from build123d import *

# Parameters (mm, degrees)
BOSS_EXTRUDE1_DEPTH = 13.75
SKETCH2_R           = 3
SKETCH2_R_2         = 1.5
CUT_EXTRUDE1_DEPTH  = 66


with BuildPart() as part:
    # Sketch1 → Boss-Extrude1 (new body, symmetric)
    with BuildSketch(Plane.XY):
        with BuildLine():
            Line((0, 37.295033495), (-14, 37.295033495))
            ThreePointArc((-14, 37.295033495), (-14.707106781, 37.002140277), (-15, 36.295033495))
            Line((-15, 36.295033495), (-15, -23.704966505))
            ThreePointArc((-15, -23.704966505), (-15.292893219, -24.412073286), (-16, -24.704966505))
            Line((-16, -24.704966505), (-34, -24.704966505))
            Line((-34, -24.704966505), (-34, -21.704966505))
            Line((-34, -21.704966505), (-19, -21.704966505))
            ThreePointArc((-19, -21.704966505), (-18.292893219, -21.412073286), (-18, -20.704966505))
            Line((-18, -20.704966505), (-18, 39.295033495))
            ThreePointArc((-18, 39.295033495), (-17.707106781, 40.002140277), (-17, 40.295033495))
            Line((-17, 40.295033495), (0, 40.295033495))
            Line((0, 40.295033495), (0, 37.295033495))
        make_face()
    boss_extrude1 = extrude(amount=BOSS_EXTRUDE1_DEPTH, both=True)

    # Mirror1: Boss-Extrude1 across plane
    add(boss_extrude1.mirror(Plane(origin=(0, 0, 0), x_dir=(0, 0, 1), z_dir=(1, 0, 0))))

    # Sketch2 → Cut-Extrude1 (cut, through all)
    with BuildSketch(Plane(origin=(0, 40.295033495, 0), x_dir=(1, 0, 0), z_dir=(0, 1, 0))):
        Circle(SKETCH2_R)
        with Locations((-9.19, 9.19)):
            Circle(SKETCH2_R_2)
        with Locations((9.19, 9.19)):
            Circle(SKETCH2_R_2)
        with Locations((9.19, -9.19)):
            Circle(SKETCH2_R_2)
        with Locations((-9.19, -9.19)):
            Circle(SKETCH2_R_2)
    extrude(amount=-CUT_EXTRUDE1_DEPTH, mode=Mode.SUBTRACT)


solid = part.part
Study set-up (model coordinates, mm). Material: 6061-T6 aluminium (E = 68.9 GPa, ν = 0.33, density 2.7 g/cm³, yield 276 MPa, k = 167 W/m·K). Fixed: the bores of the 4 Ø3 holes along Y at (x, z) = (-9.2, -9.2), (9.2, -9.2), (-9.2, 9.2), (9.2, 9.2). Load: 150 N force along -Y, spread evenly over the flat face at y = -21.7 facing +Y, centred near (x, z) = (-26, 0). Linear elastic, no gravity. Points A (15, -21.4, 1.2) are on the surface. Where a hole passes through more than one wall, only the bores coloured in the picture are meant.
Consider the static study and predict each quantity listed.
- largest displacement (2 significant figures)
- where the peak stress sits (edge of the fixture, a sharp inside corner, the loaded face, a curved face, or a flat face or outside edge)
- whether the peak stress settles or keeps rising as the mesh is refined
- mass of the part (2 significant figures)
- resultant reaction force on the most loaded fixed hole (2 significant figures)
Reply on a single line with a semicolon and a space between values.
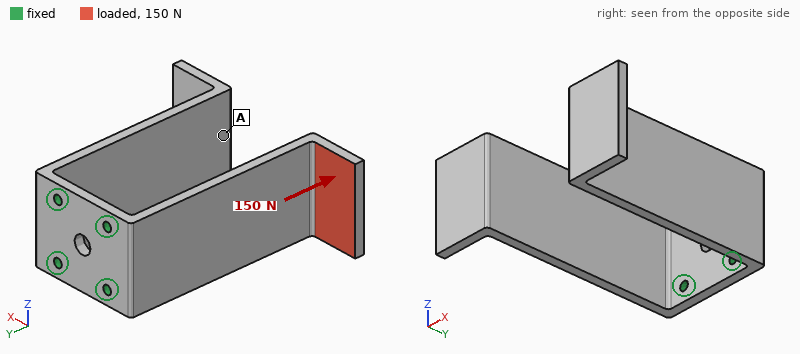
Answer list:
0.97 mm; edge of the fixture; keeps rising; 42 g; 89 N
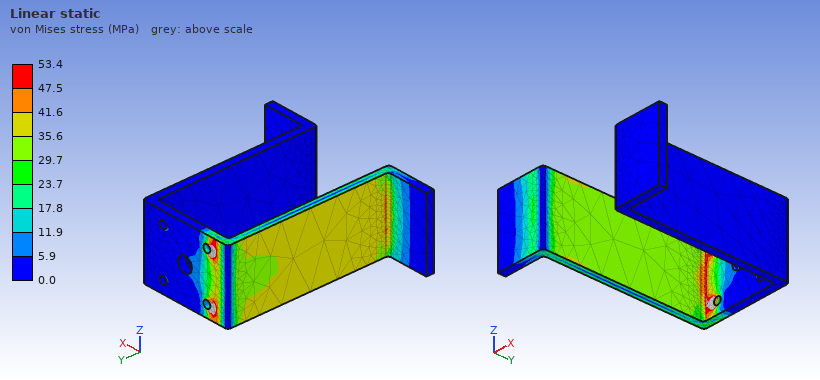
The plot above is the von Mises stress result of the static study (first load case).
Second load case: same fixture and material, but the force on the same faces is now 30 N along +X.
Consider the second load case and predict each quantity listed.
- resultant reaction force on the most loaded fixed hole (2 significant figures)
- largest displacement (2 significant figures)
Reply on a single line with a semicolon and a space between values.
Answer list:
23 N; 0.73 mm
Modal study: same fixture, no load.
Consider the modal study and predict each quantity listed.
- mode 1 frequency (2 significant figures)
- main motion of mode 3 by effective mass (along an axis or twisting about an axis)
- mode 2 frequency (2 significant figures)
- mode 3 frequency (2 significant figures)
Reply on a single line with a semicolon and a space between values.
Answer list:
380 Hz; along Z; 380 Hz; 1600 Hz
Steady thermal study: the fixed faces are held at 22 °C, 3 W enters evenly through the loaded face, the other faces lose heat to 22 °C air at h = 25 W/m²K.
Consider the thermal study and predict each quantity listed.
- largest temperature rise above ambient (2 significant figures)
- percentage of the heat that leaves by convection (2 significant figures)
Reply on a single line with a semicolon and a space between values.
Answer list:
14 K; 27 %
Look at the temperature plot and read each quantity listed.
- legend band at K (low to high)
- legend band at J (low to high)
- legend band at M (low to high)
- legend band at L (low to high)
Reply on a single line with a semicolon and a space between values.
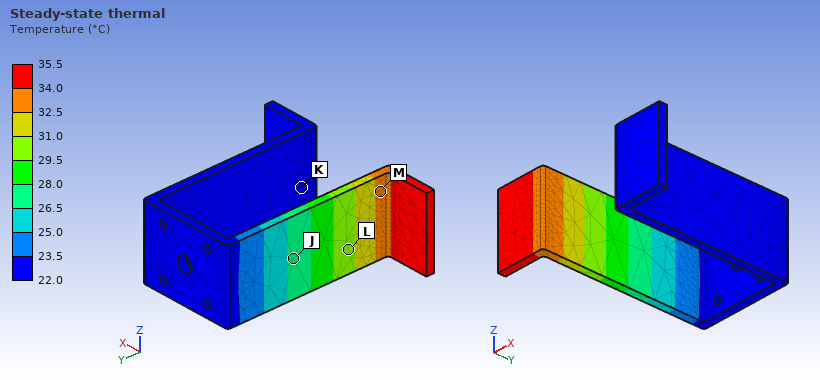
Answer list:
22.0 to 23.5 °C; 26.5 to 28.0 °C; 32.5 to 34.0 °C; 29.5 to 31.0 °C
